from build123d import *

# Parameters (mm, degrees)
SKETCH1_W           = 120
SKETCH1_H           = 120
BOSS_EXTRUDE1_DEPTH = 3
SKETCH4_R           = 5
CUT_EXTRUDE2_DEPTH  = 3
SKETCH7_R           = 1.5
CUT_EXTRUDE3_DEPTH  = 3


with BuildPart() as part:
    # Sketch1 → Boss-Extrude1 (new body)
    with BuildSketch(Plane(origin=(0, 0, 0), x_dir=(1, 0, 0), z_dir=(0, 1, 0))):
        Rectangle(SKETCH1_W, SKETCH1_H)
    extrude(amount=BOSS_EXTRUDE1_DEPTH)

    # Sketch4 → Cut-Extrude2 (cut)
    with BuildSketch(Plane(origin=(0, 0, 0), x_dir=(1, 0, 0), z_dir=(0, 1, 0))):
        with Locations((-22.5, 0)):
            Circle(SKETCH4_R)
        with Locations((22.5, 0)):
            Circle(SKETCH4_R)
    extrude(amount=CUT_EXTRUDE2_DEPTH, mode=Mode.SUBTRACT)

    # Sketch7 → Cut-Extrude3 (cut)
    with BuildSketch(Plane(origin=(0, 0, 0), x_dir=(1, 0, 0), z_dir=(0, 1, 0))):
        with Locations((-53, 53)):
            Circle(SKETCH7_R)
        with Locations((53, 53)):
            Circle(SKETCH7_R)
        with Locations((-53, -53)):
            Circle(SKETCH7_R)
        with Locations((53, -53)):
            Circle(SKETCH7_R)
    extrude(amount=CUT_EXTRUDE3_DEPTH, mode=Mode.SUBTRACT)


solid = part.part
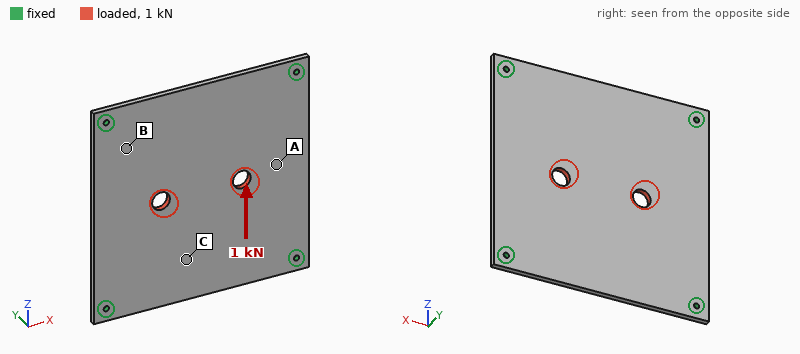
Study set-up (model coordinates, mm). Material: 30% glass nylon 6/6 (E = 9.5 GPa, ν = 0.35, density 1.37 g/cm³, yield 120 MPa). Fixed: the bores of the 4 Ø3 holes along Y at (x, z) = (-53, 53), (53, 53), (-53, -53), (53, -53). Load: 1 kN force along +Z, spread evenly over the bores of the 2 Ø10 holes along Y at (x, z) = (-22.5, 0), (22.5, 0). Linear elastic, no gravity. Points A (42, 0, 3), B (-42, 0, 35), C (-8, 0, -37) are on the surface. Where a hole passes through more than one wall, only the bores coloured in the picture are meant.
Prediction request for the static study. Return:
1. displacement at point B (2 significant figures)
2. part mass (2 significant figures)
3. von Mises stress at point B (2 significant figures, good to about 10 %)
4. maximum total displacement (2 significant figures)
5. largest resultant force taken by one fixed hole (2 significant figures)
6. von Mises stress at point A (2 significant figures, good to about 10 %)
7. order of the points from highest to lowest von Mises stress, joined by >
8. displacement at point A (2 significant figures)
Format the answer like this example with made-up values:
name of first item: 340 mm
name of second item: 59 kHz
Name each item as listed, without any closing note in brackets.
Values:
displacement at point B: 13 µm
part mass: 58 g
von Mises stress at point B: 3.4 MPa
maximum total displacement: 31 µm
largest resultant force taken by one fixed hole: 270 N
von Mises stress at point A: 2.0 MPa
order of the points from highest to lowest von Mises stress, joined by >: B > A > C
displacement at point A: 17 µm
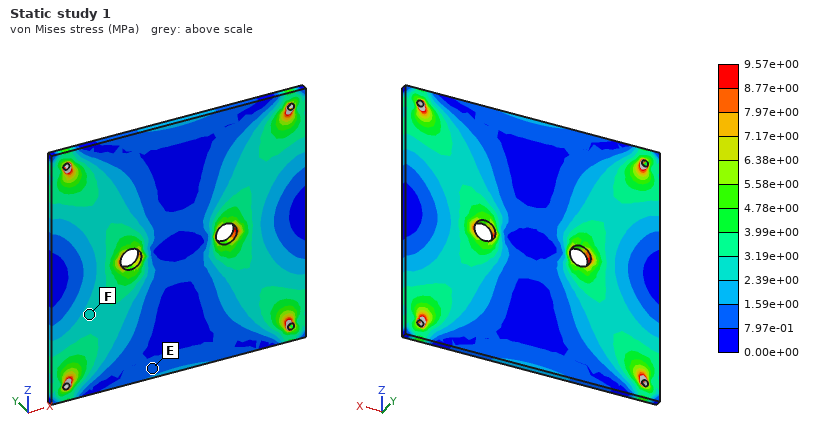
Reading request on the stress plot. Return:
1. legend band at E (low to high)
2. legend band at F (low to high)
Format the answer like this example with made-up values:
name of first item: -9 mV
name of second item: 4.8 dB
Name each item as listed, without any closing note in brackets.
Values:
legend band at E: 7.97e-01 to 1.59e+00 MPa
legend band at F: 2.39e+00 to 3.19e+00 MPa
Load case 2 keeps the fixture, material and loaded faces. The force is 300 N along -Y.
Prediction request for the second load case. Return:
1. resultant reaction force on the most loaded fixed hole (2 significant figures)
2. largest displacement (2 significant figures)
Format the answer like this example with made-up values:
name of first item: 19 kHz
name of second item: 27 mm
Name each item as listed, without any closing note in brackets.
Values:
resultant reaction force on the most loaded fixed hole: 75 N
largest displacement: 2.0 mm
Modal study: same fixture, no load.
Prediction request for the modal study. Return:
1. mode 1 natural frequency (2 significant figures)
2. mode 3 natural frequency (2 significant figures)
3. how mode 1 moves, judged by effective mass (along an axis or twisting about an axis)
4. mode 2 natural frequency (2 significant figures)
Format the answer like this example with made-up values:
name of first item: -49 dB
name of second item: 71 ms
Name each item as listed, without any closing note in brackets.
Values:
mode 1 natural frequency: 440 Hz
mode 3 natural frequency: 770 Hz
how mode 1 moves, judged by effective mass: along Y
mode 2 natural frequency: 770 Hz
